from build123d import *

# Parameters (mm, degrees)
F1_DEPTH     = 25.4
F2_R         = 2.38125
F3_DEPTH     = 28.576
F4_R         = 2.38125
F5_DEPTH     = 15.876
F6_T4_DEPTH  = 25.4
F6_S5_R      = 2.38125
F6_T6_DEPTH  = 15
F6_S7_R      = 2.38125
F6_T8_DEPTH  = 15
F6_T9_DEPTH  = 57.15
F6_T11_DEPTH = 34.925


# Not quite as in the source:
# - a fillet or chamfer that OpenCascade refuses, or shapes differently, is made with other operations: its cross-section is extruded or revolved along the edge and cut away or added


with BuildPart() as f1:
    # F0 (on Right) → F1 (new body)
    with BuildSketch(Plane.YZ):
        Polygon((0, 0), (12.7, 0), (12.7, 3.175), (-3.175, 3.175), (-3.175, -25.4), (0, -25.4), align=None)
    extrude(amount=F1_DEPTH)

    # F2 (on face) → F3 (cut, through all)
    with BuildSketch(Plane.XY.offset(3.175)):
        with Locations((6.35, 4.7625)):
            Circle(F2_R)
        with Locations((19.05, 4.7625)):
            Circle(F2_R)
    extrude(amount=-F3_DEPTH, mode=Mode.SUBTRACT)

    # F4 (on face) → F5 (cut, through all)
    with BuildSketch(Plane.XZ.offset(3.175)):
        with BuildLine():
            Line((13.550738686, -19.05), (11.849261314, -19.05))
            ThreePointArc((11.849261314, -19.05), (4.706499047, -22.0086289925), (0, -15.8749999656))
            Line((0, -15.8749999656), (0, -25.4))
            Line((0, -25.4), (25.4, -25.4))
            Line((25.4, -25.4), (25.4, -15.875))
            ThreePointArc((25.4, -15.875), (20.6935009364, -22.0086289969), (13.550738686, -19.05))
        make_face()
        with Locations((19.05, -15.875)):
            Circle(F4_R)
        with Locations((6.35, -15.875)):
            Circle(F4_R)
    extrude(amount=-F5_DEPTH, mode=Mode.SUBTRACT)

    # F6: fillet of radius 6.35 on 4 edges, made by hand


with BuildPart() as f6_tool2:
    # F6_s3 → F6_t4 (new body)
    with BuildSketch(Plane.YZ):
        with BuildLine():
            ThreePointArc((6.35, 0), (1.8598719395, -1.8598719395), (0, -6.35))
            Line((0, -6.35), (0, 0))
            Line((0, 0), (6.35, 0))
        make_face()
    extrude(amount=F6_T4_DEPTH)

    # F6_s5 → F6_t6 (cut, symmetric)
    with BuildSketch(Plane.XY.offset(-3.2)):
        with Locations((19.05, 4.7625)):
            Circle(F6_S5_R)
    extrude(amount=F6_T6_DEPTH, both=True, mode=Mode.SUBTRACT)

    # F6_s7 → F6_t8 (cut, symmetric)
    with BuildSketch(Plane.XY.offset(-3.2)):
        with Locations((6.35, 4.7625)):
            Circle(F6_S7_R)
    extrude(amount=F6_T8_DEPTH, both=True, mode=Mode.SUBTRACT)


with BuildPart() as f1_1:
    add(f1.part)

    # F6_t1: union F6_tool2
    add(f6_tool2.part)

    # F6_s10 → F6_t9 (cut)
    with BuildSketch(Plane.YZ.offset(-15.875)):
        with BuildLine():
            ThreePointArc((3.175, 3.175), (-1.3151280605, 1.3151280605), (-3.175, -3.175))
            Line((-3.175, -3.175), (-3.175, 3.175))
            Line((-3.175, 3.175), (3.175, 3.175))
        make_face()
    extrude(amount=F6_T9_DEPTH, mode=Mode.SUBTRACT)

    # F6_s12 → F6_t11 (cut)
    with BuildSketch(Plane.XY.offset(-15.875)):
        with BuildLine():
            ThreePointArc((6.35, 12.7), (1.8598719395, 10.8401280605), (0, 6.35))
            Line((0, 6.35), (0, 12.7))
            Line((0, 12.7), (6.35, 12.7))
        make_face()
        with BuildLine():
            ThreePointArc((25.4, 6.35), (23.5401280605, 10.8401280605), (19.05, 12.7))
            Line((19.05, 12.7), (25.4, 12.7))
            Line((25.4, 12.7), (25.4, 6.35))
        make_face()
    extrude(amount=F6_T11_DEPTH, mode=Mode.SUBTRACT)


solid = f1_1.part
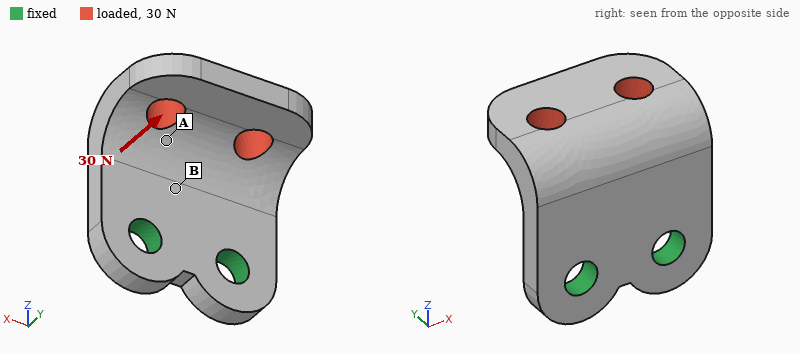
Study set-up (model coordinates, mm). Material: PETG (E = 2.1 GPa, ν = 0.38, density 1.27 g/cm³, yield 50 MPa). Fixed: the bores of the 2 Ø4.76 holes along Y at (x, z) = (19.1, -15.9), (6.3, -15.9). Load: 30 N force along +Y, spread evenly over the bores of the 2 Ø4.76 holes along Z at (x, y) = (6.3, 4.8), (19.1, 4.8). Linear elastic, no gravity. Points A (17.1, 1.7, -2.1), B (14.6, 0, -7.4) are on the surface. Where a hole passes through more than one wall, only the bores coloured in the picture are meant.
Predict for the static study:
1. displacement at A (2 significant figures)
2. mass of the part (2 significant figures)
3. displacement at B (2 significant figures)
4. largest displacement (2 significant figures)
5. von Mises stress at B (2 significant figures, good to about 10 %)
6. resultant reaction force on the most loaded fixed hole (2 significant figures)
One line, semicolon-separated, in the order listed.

0.20 mm; 3.4 g; 0.079 mm; 0.45 mm; 5.6 MPa; 15 N
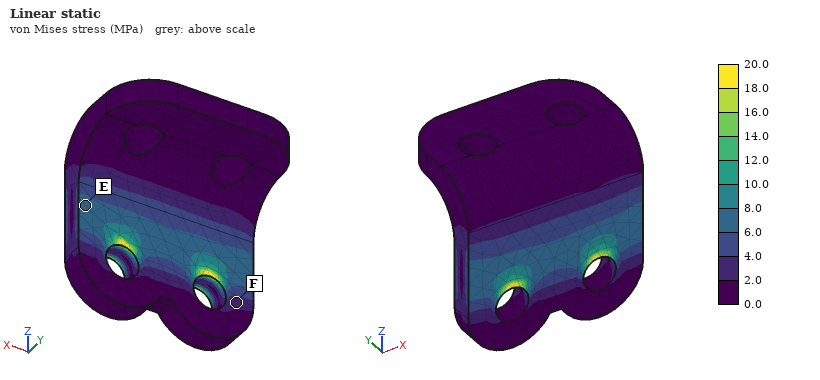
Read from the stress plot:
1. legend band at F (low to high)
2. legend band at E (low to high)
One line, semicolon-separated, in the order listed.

2.0 to 4.0 MPa; 6.0 to 8.0 MPa
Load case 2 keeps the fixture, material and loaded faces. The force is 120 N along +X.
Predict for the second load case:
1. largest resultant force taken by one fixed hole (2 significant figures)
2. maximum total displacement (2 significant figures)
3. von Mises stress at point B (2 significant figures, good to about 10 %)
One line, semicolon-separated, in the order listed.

140 N; 0.39 mm; 11 MPa
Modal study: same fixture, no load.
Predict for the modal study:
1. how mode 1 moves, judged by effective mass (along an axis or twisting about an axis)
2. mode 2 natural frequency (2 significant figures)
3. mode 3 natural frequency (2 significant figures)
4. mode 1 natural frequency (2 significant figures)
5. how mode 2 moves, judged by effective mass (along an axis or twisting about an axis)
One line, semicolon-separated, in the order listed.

along Y; 2100 Hz; 4100 Hz; 1100 Hz; along X
